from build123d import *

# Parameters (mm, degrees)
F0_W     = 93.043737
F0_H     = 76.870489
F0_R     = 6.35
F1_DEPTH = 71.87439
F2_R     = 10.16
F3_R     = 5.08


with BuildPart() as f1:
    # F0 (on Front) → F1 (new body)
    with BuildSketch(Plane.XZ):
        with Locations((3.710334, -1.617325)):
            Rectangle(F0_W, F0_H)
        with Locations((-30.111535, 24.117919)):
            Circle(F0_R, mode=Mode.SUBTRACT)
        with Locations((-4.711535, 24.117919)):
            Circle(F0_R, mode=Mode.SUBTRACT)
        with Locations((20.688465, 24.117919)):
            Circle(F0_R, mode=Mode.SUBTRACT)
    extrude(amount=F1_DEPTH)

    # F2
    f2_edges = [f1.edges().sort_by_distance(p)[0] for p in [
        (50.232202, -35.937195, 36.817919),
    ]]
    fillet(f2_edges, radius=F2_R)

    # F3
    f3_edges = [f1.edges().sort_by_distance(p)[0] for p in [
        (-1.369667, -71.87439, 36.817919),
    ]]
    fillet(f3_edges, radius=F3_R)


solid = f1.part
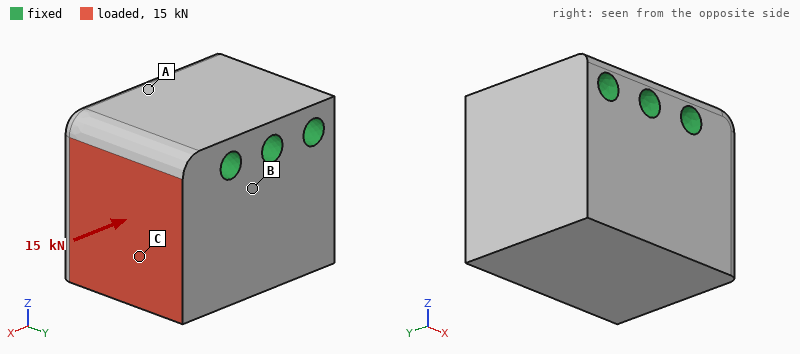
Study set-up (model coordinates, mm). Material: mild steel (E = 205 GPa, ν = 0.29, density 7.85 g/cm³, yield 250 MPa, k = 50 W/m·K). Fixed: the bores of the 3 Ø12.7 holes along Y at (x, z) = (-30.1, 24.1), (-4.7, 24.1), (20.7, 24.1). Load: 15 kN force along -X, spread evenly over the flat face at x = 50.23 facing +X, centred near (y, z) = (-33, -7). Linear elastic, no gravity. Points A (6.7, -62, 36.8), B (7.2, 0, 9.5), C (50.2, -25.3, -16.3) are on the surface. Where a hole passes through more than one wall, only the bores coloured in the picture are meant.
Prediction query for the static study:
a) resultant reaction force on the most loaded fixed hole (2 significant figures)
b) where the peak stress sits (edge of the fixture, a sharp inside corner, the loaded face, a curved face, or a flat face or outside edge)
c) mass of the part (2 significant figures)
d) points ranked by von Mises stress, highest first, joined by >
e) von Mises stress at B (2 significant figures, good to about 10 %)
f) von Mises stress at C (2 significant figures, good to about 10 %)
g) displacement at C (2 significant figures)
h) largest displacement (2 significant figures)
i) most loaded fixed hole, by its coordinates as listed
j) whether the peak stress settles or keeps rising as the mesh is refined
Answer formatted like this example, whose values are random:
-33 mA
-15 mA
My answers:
11 kN
edge of the fixture
3.8 kg
B > C > A
5.8 MPa
3.0 MPa
2.4 µm
3.1 µm
(20.7, 24.1)
keeps rising
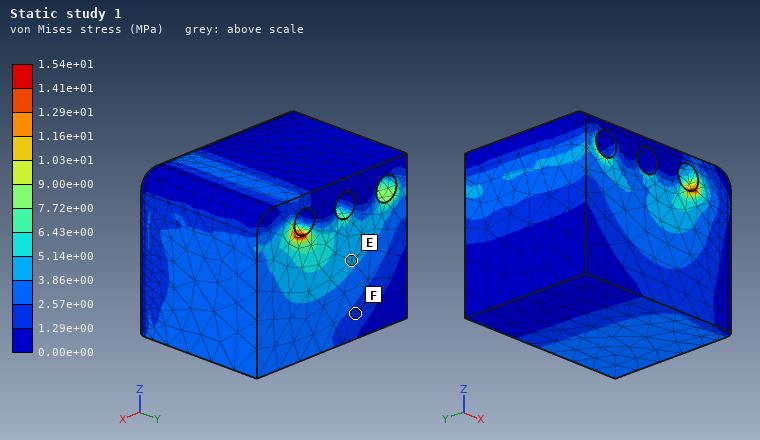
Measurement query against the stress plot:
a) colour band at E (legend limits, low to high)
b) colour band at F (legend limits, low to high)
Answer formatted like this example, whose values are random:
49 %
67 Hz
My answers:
3.86e+00 to 5.14e+00 MPa
1.29e+00 to 2.57e+00 MPa
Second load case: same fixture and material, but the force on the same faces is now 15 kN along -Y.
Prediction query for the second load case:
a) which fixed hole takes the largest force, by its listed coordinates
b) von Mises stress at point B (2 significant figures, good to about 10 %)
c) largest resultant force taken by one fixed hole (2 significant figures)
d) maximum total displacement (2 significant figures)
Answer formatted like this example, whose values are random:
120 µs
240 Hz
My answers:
(20.7, 24.1)
9.1 MPa
14 kN
5.9 µm
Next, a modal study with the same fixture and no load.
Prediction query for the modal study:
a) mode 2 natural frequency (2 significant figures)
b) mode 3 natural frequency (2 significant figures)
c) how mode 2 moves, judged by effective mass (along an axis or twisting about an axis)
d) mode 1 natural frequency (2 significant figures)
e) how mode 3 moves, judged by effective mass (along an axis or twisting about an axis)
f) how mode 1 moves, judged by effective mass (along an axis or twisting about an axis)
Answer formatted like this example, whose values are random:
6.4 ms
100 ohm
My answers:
8900 Hz
12 kHz
along Y
8400 Hz
twisting about Z
along X
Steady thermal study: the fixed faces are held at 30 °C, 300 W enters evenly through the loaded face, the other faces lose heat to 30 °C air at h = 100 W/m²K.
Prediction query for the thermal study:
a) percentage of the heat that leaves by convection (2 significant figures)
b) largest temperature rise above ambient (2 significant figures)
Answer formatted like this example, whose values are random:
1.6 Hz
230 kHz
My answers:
14 %
60 K
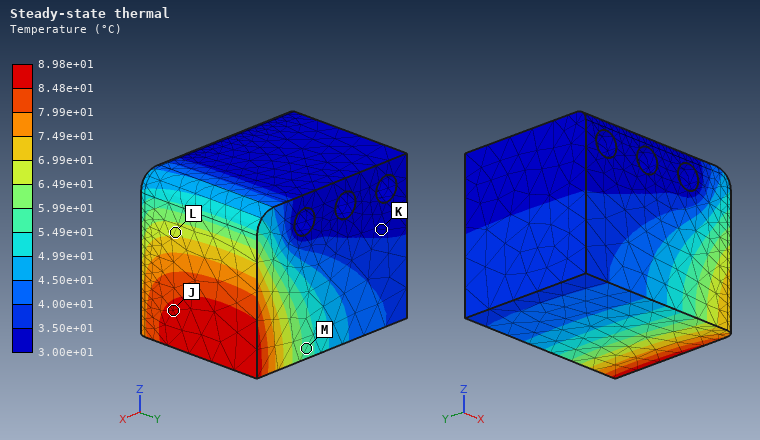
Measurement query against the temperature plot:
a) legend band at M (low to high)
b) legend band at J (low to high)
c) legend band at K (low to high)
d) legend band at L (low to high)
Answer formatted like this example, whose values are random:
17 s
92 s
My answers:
5.49e+01 to 5.99e+01 °C
8.48e+01 to 8.98e+01 °C
3.00e+01 to 3.50e+01 °C
6.49e+01 to 6.99e+01 °C
